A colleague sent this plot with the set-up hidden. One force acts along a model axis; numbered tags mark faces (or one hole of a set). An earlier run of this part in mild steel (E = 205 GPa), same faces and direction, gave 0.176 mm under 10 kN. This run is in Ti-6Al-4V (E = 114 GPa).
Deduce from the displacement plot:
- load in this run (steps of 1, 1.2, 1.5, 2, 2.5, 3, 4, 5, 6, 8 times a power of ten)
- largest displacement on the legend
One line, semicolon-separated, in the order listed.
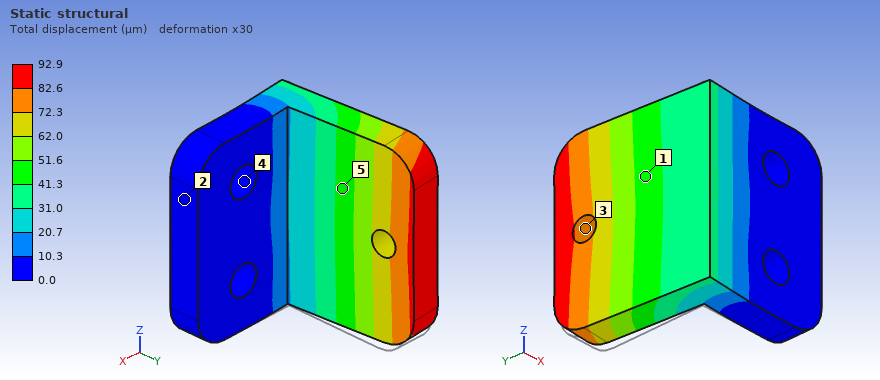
3 kN; 92.9 µm
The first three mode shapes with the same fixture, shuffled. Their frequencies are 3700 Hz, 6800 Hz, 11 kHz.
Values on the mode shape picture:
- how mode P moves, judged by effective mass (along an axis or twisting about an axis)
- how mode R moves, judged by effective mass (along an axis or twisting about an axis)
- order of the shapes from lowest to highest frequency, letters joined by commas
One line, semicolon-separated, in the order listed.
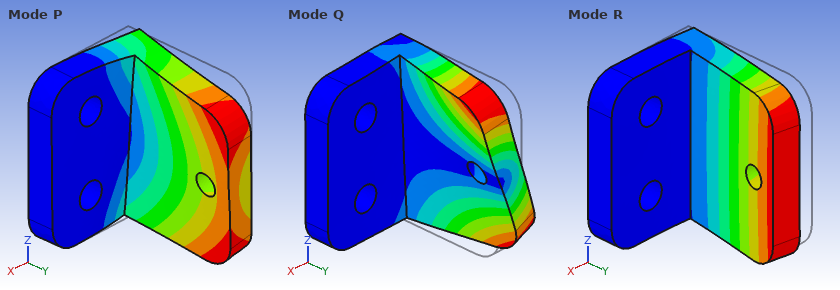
along Z; along X; R, P, Q
